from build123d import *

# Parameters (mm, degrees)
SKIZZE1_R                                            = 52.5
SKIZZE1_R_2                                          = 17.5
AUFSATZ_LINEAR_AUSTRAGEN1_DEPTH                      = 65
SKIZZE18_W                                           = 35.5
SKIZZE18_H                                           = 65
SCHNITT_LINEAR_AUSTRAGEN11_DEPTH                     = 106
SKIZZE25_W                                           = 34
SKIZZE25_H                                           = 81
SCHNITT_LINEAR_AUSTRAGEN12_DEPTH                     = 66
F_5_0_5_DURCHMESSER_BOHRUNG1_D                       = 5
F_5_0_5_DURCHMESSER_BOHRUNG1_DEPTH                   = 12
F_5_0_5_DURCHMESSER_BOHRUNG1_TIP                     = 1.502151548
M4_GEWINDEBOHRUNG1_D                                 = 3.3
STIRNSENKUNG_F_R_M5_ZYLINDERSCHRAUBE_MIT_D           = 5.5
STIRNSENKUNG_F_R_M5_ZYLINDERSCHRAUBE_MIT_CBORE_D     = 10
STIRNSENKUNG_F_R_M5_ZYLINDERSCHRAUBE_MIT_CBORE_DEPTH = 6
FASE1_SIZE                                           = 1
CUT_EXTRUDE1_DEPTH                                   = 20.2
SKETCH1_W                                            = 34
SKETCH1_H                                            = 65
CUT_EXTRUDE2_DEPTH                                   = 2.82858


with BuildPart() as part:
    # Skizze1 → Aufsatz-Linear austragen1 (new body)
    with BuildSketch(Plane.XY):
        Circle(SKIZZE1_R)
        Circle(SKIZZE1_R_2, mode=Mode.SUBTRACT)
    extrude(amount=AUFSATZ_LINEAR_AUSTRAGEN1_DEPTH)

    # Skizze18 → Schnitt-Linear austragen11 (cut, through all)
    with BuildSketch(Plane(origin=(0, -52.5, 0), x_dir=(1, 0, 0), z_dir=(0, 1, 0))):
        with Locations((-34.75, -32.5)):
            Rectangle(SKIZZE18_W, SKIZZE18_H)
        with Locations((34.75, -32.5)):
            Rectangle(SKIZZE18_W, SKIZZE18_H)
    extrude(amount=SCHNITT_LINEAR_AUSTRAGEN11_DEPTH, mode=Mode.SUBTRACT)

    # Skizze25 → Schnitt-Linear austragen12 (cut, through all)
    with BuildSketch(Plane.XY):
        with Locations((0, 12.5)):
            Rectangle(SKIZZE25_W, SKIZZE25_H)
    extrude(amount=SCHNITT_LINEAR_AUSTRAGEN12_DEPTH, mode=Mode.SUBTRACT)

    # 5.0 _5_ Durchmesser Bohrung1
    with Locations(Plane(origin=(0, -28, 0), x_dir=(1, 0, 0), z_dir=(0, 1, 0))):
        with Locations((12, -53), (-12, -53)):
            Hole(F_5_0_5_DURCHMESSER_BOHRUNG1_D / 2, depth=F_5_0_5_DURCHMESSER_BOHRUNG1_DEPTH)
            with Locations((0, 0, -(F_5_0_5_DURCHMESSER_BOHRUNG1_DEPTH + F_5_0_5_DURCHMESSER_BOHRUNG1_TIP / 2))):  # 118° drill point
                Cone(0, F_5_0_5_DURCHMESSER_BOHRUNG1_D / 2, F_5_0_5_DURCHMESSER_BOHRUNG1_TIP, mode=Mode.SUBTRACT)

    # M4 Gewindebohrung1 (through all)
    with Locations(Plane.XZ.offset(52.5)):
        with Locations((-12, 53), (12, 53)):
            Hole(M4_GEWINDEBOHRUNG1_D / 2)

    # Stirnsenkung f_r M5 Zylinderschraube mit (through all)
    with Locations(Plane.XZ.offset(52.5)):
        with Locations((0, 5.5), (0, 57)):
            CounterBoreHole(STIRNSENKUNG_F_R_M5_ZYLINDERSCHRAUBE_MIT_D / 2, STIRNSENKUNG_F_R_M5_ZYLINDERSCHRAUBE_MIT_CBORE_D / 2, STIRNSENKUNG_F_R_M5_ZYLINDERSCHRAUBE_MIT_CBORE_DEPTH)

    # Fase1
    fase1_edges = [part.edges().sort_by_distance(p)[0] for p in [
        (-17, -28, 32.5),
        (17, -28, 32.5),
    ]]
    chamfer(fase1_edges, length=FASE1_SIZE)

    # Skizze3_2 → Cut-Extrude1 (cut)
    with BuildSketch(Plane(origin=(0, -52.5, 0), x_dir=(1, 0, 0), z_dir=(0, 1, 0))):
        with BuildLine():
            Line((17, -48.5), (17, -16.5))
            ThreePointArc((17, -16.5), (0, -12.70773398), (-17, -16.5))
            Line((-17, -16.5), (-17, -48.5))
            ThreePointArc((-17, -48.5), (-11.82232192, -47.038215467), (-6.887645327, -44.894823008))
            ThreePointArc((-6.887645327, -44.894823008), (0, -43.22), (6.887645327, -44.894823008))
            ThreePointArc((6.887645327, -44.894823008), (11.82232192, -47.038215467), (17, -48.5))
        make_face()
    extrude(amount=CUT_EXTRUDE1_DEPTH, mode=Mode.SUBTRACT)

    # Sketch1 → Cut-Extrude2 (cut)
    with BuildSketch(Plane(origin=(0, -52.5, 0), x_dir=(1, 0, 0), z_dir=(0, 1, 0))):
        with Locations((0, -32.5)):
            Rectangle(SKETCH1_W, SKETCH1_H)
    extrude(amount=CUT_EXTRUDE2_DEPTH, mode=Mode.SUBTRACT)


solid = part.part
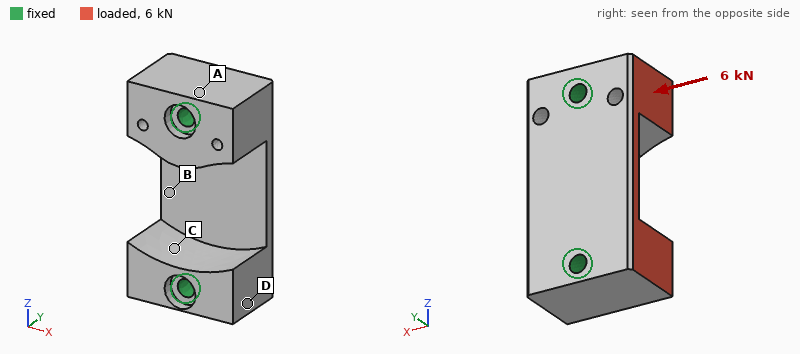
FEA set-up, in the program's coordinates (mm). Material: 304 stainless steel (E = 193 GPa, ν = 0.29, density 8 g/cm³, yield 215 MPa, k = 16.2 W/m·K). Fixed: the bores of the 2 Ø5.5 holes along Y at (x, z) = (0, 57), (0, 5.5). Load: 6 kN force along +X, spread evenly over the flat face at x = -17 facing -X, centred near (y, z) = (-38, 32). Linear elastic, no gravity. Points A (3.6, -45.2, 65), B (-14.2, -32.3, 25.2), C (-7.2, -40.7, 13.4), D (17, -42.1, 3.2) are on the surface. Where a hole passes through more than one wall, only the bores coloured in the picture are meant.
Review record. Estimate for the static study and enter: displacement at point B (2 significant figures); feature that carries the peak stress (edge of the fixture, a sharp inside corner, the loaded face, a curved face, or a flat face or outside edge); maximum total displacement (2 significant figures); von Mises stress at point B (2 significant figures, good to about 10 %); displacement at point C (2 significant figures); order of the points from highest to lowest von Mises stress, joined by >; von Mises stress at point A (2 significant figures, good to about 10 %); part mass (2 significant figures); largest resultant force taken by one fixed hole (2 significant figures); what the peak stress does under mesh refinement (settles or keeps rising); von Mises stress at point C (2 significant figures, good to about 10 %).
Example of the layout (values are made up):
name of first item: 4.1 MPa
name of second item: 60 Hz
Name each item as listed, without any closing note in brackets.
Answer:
displacement at point B: 1.7 µm
feature that carries the peak stress: edge of the fixture
maximum total displacement: 2.9 µm
von Mises stress at point B: 9.3 MPa
displacement at point C: 1.1 µm
order of the points from highest to lowest von Mises stress, joined by >: C > B > A > D
von Mises stress at point A: 5.0 MPa
part mass: 220 g
largest resultant force taken by one fixed hole: 3.1 kN
what the peak stress does under mesh refinement: keeps rising
von Mises stress at point C: 16 MPa
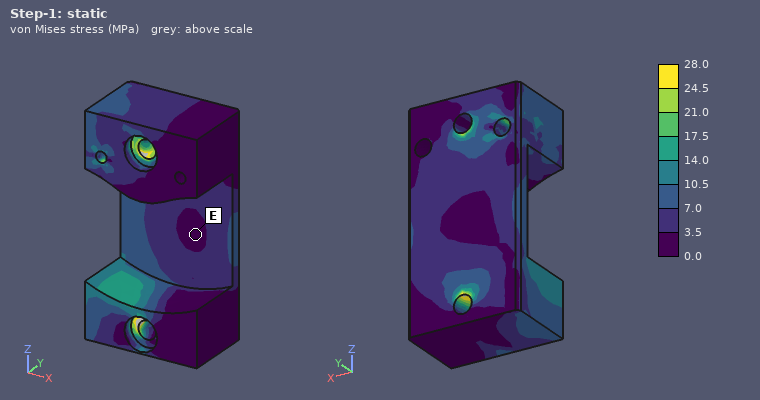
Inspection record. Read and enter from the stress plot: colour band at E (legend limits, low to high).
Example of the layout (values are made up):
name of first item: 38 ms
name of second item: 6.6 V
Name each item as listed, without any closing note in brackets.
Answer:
colour band at E: 0.0 to 3.5 MPa
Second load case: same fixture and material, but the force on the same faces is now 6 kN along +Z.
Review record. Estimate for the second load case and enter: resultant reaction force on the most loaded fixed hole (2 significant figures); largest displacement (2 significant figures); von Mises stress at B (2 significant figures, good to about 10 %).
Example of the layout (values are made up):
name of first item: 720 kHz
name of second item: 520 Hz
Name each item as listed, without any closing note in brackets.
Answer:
resultant reaction force on the most loaded fixed hole: 3.4 kN
largest displacement: 10 µm
von Mises stress at B: 21 MPa
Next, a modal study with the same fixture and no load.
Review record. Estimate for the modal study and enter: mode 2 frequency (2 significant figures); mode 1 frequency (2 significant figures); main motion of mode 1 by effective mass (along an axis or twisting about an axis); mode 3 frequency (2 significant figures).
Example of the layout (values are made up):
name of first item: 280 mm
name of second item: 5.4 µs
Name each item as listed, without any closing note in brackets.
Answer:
mode 2 frequency: 16 kHz
mode 1 frequency: 15 kHz
main motion of mode 1 by effective mass: along Y
mode 3 frequency: 19 kHz
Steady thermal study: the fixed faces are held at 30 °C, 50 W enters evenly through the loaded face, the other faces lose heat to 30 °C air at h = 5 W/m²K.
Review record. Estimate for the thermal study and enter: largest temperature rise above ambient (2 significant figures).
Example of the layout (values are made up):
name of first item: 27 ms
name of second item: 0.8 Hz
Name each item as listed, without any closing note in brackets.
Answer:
largest temperature rise above ambient: 86 K
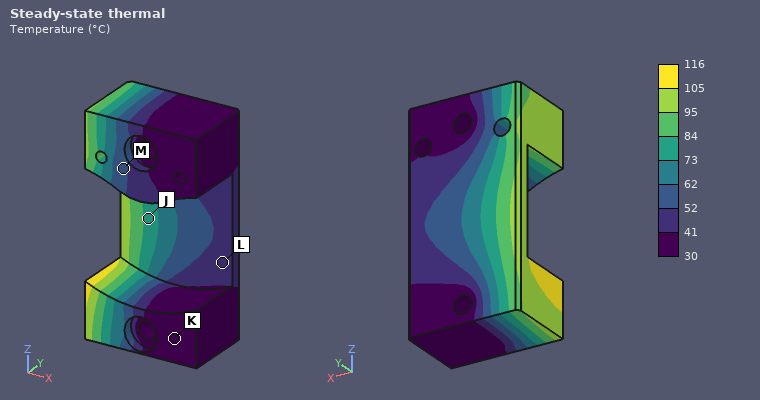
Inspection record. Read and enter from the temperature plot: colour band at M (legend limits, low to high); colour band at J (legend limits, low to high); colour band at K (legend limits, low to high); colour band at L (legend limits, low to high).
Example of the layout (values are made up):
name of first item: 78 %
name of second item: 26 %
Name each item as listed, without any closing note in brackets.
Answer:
colour band at M: 52 to 62 °C
colour band at J: 73 to 84 °C
colour band at K: 30 to 41 °C
colour band at L: 41 to 52 °C
